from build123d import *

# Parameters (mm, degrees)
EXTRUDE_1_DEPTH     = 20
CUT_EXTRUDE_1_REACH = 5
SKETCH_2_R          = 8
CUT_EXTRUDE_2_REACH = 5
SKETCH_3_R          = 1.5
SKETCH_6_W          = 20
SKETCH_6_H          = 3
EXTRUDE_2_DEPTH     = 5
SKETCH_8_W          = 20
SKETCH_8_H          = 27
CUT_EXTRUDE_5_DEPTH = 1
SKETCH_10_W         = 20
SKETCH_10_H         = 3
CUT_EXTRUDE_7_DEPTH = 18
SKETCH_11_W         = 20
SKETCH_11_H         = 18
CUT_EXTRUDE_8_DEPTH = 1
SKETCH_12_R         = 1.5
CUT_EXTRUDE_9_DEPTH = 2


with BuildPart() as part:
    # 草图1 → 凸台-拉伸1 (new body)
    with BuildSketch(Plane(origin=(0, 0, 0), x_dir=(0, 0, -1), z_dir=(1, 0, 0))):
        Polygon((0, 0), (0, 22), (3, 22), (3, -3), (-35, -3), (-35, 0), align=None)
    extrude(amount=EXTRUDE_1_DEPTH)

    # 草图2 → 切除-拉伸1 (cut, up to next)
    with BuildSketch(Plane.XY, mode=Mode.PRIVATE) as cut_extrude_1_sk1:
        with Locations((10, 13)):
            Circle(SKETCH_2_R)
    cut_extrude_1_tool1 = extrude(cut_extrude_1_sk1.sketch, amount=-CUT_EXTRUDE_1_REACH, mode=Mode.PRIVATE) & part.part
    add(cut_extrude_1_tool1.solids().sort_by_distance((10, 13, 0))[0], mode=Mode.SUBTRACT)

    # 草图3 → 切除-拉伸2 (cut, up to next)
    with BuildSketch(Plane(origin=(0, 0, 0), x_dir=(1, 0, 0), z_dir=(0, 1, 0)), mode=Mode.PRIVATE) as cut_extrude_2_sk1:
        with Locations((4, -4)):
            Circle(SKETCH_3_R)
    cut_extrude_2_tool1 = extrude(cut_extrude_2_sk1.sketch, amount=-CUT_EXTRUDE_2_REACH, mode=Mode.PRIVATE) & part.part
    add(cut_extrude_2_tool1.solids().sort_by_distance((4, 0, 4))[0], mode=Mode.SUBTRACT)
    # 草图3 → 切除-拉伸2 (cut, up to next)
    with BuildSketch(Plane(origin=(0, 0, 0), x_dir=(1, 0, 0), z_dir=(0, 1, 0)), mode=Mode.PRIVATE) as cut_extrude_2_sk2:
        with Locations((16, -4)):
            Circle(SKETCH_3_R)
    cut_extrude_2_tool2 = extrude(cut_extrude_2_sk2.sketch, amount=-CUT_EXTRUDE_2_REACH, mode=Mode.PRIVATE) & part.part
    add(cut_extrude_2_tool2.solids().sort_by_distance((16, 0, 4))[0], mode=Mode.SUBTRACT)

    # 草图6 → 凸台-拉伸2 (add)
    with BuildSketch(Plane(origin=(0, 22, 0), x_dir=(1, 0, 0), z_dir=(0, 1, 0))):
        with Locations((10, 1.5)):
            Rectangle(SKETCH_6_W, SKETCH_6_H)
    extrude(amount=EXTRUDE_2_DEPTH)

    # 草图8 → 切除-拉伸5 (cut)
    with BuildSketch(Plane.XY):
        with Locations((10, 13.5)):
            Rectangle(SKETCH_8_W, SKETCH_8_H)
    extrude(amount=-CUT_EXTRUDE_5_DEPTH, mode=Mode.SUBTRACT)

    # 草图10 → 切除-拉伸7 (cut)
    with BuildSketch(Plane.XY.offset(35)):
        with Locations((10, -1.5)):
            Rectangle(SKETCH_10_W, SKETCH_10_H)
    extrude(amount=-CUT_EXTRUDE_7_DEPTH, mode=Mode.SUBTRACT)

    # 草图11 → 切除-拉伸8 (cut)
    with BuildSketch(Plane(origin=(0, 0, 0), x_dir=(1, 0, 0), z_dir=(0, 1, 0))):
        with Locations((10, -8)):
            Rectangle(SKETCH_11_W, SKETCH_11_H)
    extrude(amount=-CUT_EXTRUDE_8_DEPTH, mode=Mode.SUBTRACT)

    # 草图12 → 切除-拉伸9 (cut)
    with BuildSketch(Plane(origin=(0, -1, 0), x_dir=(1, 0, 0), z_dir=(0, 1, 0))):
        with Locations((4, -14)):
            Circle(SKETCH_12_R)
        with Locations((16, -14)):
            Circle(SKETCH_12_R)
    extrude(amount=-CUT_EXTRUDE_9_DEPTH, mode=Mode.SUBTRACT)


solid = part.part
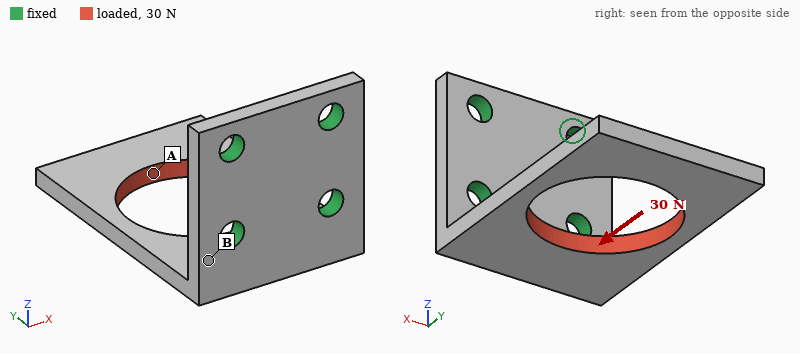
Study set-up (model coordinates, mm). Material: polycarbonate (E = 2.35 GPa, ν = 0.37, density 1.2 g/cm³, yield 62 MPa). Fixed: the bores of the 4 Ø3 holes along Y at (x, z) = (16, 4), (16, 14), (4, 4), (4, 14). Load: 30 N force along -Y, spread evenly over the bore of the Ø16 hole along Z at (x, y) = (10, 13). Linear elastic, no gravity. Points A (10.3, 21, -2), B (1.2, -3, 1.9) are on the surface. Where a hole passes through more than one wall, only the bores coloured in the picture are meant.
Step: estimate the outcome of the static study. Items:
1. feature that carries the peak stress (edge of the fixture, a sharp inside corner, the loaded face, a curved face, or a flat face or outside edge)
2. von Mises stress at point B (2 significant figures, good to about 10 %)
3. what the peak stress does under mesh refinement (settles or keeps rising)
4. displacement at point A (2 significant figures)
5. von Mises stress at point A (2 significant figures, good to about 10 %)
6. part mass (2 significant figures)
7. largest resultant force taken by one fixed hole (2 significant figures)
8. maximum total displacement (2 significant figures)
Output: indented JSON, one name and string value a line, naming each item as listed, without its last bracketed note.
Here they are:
{
  "feature that carries the peak stress": "edge of the fixture",
  "von Mises stress at point B": "6.7 MPa",
  "what the peak stress does under mesh refinement": "keeps rising",
  "displacement at point A": "0.31 mm",
  "von Mises stress at point A": "1.9 MPa",
  "part mass": "1.8 g",
  "largest resultant force taken by one fixed hole": "16 N",
  "maximum total displacement": "0.38 mm"
}
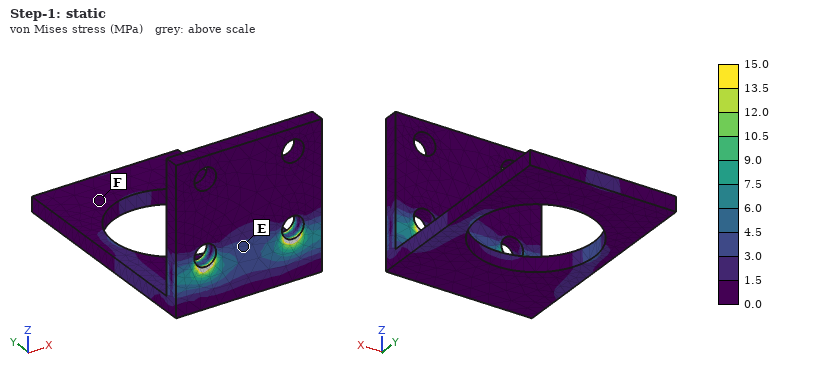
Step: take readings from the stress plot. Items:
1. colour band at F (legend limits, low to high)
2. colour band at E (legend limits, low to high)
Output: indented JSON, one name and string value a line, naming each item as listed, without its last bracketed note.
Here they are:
{
  "colour band at F": "0.0 to 1.5 MPa",
  "colour band at E": "3.0 to 4.5 MPa"
}
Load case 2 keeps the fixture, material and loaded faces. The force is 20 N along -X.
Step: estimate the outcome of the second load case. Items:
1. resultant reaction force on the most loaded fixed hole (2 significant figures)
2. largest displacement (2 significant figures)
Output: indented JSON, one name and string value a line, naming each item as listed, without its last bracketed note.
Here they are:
{
  "resultant reaction force on the most loaded fixed hole": "26 N",
  "largest displacement": "0.40 mm"
}
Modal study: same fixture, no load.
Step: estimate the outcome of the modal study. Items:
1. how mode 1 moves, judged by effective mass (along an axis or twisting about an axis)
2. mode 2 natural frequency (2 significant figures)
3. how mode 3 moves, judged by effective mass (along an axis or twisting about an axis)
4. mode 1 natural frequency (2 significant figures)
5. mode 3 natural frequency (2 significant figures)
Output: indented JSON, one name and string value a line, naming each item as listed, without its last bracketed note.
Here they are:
{
  "how mode 1 moves, judged by effective mass": "along Z",
  "mode 2 natural frequency": "1200 Hz",
  "how mode 3 moves, judged by effective mass": "along X",
  "mode 1 natural frequency": "390 Hz",
  "mode 3 natural frequency": "1500 Hz"
}
